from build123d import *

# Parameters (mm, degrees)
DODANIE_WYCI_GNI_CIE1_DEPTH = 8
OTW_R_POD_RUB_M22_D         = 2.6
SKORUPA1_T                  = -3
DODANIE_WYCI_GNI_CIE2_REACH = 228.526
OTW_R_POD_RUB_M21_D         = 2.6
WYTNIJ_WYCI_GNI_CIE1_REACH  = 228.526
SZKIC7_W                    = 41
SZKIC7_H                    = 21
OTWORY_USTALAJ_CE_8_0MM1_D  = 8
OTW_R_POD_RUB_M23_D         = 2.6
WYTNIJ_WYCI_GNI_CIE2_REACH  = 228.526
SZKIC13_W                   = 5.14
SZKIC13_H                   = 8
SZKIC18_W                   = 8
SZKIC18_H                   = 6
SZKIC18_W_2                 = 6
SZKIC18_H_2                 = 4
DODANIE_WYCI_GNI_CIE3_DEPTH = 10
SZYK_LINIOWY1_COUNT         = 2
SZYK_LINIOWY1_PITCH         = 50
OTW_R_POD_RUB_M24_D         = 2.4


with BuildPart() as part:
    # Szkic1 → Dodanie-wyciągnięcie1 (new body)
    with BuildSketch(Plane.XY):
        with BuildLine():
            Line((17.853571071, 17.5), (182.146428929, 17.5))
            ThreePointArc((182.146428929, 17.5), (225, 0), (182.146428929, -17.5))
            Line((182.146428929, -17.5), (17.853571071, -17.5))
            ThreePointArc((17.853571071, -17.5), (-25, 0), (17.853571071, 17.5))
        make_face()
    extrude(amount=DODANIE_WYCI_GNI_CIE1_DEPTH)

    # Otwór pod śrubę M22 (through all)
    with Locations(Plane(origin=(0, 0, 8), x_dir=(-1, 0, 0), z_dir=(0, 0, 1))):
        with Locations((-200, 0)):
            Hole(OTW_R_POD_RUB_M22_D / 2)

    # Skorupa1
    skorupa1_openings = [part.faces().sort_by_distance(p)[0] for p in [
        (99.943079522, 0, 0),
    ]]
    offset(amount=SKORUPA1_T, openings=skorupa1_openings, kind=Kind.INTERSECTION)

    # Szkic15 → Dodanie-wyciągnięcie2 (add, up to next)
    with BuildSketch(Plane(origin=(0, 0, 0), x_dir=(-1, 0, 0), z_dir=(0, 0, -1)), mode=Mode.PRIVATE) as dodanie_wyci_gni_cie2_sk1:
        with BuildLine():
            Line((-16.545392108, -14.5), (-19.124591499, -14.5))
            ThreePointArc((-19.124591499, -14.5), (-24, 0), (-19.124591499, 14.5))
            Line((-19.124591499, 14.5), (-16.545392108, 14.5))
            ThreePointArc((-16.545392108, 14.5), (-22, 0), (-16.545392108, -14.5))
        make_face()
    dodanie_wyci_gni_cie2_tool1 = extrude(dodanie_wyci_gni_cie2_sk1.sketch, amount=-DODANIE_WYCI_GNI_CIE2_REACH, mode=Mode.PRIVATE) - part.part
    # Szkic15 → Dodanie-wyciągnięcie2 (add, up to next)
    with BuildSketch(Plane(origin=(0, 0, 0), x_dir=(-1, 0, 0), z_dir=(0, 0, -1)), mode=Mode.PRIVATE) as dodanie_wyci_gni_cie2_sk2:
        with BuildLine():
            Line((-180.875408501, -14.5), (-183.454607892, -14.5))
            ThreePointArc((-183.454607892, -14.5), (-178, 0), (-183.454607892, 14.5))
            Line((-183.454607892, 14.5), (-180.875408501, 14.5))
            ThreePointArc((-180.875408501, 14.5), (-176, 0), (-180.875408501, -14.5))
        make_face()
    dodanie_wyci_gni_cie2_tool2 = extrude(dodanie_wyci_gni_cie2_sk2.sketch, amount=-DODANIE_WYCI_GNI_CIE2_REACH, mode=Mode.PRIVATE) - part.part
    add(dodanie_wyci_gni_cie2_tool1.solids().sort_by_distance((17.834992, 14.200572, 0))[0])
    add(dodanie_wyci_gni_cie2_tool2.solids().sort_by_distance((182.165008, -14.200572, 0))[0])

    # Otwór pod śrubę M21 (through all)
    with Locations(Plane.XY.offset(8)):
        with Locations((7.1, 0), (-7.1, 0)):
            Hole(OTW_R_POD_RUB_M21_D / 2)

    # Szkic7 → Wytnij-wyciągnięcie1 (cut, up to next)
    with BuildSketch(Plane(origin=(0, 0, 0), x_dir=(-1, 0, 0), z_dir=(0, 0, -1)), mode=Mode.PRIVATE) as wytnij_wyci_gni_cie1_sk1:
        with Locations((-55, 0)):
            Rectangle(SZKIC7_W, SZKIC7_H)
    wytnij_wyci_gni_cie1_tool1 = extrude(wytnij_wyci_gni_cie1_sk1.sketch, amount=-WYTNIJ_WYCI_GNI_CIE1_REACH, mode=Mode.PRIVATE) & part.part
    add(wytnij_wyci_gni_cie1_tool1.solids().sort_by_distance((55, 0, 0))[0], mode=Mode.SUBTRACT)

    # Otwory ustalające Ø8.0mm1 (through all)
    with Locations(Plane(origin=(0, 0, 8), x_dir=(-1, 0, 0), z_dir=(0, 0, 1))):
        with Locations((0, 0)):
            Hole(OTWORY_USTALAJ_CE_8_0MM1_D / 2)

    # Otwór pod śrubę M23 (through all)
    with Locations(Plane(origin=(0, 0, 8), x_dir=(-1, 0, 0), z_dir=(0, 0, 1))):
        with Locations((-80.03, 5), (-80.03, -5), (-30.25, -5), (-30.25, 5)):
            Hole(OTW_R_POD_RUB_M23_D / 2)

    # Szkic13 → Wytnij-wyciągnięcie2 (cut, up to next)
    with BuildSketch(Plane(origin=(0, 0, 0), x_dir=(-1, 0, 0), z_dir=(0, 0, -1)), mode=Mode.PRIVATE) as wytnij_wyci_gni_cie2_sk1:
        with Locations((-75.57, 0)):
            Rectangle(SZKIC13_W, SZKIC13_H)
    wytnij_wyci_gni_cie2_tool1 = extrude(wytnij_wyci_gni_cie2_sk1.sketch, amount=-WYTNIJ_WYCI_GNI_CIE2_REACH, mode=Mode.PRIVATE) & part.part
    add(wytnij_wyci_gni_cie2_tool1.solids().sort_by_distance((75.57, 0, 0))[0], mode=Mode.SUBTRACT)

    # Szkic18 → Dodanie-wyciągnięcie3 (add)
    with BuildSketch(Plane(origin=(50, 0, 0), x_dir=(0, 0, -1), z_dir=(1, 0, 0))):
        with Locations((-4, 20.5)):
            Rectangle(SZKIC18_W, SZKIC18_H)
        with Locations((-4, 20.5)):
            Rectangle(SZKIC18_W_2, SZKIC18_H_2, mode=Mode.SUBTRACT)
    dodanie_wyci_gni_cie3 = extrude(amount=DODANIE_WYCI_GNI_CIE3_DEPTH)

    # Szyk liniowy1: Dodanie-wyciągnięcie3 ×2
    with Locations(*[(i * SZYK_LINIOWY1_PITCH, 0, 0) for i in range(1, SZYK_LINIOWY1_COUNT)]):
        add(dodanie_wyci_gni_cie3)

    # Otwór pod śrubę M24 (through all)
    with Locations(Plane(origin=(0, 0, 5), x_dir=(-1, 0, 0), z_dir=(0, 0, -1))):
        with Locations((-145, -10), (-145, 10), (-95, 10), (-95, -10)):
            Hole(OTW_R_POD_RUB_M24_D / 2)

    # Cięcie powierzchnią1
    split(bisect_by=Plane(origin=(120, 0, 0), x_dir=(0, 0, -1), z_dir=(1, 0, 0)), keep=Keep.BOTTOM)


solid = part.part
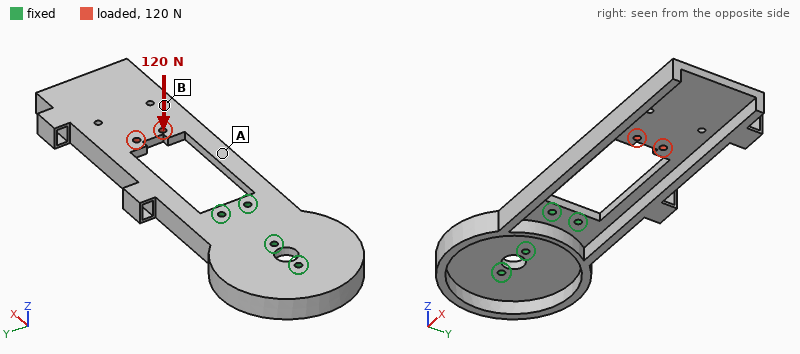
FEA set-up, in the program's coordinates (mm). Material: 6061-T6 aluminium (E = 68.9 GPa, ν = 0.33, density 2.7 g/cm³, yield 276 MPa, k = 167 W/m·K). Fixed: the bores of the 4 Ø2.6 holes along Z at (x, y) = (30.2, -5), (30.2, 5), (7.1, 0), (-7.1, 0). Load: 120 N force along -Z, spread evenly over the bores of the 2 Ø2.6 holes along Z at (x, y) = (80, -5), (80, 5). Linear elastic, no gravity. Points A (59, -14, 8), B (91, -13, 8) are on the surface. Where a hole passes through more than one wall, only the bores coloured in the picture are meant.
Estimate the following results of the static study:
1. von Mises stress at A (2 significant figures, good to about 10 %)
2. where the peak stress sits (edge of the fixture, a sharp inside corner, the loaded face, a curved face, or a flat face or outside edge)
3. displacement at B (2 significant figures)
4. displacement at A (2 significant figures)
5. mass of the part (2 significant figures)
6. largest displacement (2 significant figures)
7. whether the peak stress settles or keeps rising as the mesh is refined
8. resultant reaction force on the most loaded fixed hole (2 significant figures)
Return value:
23 MPa
edge of the fixture
0.44 mm
0.17 mm
51 g
0.68 mm
keeps rising
170 N
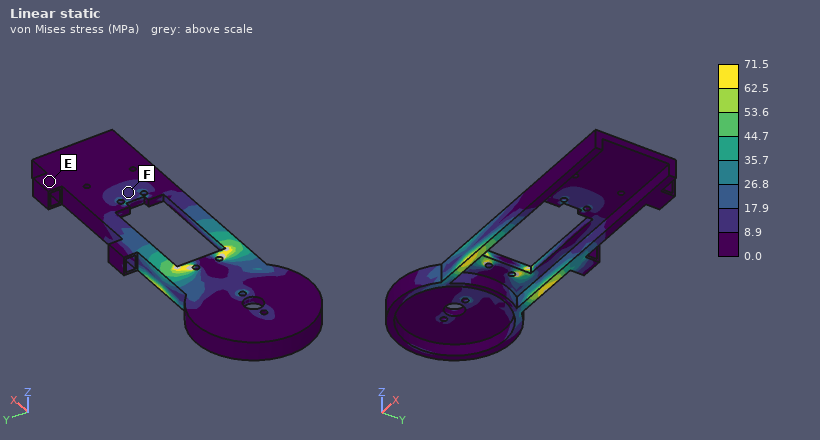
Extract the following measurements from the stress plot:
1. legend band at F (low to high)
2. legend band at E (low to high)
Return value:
8.9 to 17.9 MPa
0.0 to 8.9 MPa
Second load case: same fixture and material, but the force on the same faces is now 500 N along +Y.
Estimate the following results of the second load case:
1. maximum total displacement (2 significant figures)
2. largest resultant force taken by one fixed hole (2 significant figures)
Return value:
0.48 mm
650 N
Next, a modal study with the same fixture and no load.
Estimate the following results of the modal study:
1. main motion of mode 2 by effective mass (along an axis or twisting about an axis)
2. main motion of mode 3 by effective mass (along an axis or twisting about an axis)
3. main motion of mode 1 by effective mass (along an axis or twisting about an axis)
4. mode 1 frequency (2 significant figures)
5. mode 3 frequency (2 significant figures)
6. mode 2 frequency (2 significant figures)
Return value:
along Y
along Y
along Z
470 Hz
1400 Hz
1000 Hz
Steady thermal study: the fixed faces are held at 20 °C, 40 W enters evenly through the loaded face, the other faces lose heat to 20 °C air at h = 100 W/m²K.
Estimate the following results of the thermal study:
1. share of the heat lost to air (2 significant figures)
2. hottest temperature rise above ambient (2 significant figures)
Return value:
79 %
79 K
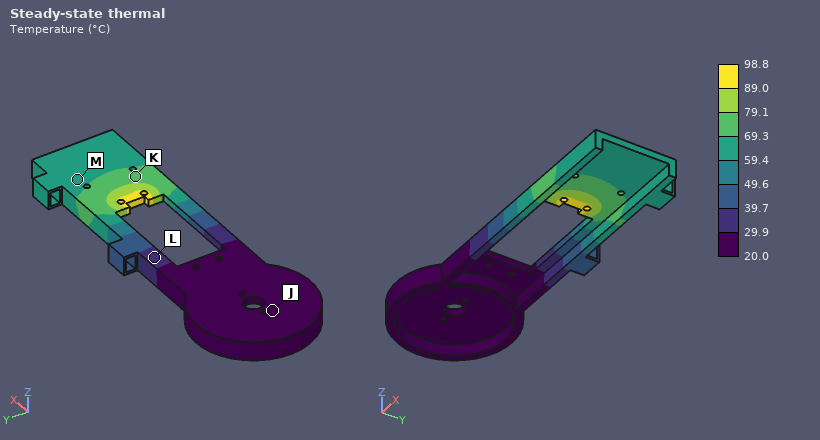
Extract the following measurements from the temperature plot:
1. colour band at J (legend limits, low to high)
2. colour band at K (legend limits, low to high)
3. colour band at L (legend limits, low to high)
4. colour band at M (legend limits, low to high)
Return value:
20.0 to 29.9 °C
69.3 to 79.1 °C
29.9 to 39.7 °C
59.4 to 69.3 °C
